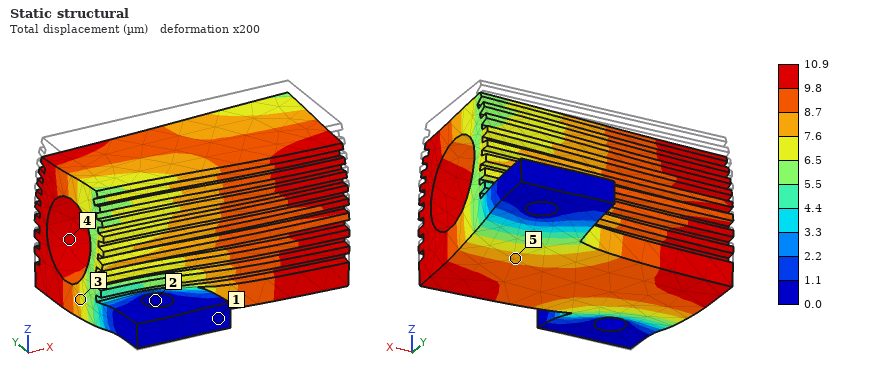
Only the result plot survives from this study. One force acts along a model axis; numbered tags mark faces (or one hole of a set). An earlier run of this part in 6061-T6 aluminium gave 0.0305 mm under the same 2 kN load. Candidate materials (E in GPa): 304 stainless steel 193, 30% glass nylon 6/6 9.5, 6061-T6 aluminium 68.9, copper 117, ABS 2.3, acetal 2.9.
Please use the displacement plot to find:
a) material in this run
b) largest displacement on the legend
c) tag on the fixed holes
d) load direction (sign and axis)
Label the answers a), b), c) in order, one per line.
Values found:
a) 304 stainless steel
b) 10.9 µm
c) 2
d) -Z
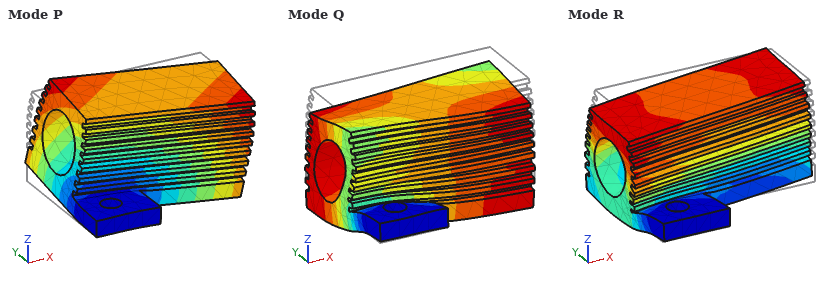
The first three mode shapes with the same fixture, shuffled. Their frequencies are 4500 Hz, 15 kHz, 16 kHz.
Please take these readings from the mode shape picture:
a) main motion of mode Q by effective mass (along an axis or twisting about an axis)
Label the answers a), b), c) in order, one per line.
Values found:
a) along Z
